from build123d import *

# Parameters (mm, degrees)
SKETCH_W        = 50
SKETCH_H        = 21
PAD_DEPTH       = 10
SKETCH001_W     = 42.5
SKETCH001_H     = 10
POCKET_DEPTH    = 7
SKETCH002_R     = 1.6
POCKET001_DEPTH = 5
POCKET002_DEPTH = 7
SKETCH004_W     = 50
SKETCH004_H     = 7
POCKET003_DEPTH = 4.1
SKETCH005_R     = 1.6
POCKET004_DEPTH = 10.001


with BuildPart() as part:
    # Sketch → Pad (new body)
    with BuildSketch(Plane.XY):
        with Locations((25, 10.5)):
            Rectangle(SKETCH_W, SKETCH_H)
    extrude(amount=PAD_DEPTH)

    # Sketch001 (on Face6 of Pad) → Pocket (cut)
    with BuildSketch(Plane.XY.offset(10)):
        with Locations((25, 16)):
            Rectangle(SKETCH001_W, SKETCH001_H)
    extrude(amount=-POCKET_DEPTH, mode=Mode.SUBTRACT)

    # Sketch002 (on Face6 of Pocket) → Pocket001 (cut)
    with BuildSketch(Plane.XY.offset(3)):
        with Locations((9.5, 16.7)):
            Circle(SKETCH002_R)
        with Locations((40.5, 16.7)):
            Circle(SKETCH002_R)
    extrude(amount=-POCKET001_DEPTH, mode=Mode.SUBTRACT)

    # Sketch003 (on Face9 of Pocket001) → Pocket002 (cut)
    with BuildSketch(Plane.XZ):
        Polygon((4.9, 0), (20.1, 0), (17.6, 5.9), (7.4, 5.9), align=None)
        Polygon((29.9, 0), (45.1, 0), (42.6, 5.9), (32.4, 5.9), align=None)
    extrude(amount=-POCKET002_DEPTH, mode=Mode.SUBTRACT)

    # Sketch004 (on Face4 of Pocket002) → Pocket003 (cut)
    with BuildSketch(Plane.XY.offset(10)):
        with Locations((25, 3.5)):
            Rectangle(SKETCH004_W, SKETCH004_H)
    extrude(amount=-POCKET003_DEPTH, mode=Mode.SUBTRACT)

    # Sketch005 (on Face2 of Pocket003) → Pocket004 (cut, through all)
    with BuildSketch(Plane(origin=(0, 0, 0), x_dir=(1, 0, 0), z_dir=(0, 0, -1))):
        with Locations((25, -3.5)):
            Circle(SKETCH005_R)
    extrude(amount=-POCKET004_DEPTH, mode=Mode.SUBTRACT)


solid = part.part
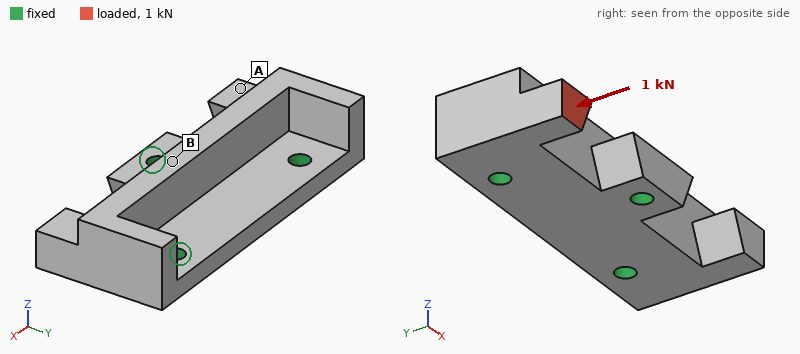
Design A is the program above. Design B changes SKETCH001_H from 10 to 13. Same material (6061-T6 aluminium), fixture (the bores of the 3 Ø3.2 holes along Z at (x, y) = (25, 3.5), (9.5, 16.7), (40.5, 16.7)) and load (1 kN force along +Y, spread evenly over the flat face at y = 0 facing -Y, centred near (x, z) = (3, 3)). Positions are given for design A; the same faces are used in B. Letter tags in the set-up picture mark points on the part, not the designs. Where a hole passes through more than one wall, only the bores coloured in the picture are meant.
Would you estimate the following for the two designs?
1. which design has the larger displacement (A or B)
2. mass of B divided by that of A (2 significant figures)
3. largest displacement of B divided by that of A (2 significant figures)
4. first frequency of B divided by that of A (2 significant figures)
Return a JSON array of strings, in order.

["B", "0.91", "1.2", "0.93"]
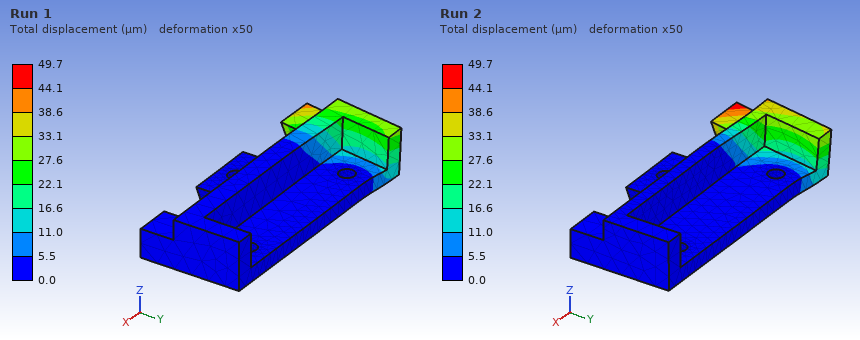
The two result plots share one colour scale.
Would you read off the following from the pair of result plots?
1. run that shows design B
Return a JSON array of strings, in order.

["Run 2"]
